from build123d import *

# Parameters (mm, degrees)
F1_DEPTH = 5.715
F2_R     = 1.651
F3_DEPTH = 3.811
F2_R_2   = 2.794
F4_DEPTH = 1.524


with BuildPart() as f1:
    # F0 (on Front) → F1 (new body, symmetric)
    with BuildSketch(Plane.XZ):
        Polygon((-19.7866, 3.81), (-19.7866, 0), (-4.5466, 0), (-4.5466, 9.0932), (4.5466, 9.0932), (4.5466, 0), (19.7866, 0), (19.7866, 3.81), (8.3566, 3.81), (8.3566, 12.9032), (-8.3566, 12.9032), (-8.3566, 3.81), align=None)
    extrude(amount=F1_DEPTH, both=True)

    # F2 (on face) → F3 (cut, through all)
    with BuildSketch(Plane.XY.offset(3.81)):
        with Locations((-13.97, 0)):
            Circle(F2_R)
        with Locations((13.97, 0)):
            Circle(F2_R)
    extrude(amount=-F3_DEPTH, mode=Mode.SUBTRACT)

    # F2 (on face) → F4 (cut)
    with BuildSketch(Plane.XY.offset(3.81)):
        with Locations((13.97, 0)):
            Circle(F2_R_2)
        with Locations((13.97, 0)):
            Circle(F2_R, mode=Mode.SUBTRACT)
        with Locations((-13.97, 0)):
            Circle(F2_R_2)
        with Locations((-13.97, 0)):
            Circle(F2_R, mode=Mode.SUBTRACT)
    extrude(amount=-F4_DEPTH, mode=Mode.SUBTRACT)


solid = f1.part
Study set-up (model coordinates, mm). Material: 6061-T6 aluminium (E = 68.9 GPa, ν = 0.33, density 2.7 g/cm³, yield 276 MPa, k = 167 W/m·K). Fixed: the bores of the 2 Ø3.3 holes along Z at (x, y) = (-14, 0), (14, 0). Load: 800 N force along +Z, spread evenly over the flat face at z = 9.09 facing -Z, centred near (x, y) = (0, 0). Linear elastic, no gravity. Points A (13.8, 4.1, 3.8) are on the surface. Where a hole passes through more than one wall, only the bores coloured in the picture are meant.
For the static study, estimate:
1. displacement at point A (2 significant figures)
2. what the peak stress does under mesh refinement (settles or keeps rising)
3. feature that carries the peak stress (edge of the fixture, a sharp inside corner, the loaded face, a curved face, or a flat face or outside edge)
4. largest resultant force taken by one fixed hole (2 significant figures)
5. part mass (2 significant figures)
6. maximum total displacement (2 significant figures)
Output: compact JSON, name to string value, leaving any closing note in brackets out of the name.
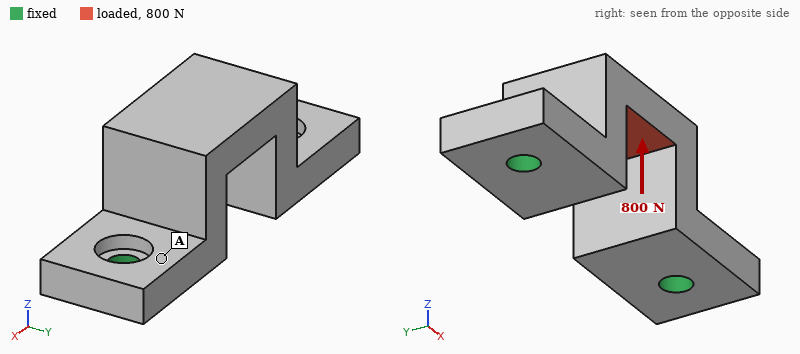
{"displacement at point A": "2.4 µm", "what the peak stress does under mesh refinement": "keeps rising", "feature that carries the peak stress": "edge of the fixture", "largest resultant force taken by one fixed hole": "500 N", "part mass": "6.5 g", "maximum total displacement": "13 µm"}
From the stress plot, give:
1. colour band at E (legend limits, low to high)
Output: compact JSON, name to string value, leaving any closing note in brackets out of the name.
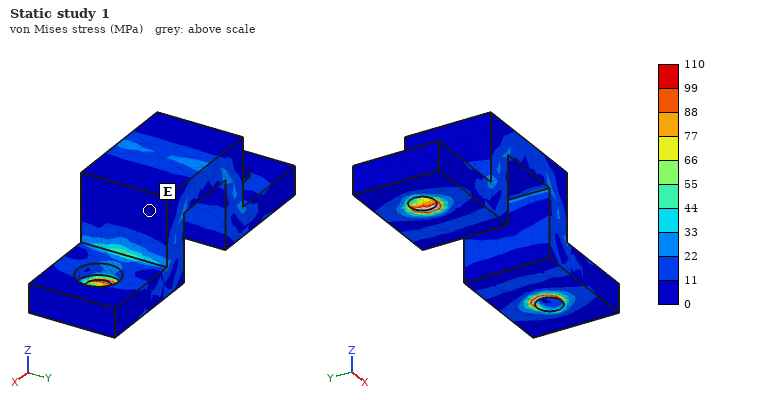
{"colour band at E": "0 to 11 MPa"}
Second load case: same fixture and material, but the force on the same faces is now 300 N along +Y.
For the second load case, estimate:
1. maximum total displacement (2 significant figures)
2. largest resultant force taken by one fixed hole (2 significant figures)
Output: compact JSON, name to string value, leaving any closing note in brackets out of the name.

{"maximum total displacement": "33 µm", "largest resultant force taken by one fixed hole": "150 N"}
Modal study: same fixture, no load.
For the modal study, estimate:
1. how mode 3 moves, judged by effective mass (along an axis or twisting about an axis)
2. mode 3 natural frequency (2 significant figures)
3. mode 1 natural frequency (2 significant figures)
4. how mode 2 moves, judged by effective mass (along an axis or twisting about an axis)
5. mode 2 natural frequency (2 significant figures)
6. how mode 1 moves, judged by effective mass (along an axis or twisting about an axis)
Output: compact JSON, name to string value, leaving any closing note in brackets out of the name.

{"how mode 3 moves, judged by effective mass": "along X", "mode 3 natural frequency": "23 kHz", "mode 1 natural frequency": "9100 Hz", "how mode 2 moves, judged by effective mass": "along Z", "mode 2 natural frequency": "21 kHz", "how mode 1 moves, judged by effective mass": "along Y"}
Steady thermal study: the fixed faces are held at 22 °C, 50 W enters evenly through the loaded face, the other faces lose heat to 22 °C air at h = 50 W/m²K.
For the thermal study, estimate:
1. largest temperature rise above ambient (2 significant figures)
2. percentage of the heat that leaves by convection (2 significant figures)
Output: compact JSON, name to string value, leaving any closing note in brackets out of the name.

{"largest temperature rise above ambient": "65 K", "percentage of the heat that leaves by convection": "4.7 %"}
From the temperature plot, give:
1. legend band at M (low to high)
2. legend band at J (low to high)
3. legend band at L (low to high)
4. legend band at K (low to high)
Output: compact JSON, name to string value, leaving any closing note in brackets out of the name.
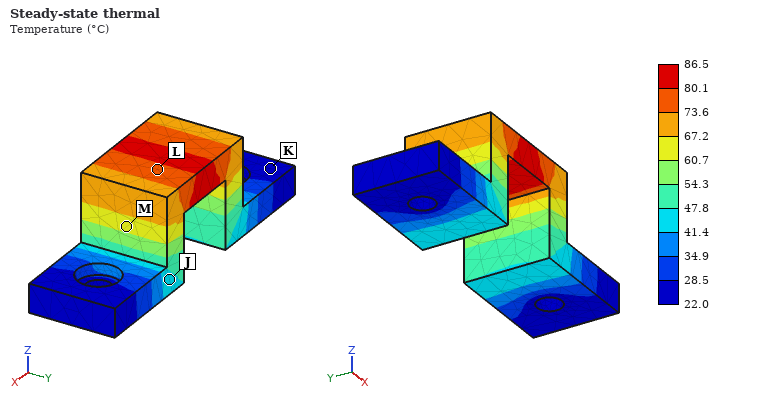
{"legend band at M": "60.7 to 67.2 °C", "legend band at J": "41.4 to 47.8 °C", "legend band at L": "73.6 to 80.1 °C", "legend band at K": "22.0 to 28.5 °C"}
